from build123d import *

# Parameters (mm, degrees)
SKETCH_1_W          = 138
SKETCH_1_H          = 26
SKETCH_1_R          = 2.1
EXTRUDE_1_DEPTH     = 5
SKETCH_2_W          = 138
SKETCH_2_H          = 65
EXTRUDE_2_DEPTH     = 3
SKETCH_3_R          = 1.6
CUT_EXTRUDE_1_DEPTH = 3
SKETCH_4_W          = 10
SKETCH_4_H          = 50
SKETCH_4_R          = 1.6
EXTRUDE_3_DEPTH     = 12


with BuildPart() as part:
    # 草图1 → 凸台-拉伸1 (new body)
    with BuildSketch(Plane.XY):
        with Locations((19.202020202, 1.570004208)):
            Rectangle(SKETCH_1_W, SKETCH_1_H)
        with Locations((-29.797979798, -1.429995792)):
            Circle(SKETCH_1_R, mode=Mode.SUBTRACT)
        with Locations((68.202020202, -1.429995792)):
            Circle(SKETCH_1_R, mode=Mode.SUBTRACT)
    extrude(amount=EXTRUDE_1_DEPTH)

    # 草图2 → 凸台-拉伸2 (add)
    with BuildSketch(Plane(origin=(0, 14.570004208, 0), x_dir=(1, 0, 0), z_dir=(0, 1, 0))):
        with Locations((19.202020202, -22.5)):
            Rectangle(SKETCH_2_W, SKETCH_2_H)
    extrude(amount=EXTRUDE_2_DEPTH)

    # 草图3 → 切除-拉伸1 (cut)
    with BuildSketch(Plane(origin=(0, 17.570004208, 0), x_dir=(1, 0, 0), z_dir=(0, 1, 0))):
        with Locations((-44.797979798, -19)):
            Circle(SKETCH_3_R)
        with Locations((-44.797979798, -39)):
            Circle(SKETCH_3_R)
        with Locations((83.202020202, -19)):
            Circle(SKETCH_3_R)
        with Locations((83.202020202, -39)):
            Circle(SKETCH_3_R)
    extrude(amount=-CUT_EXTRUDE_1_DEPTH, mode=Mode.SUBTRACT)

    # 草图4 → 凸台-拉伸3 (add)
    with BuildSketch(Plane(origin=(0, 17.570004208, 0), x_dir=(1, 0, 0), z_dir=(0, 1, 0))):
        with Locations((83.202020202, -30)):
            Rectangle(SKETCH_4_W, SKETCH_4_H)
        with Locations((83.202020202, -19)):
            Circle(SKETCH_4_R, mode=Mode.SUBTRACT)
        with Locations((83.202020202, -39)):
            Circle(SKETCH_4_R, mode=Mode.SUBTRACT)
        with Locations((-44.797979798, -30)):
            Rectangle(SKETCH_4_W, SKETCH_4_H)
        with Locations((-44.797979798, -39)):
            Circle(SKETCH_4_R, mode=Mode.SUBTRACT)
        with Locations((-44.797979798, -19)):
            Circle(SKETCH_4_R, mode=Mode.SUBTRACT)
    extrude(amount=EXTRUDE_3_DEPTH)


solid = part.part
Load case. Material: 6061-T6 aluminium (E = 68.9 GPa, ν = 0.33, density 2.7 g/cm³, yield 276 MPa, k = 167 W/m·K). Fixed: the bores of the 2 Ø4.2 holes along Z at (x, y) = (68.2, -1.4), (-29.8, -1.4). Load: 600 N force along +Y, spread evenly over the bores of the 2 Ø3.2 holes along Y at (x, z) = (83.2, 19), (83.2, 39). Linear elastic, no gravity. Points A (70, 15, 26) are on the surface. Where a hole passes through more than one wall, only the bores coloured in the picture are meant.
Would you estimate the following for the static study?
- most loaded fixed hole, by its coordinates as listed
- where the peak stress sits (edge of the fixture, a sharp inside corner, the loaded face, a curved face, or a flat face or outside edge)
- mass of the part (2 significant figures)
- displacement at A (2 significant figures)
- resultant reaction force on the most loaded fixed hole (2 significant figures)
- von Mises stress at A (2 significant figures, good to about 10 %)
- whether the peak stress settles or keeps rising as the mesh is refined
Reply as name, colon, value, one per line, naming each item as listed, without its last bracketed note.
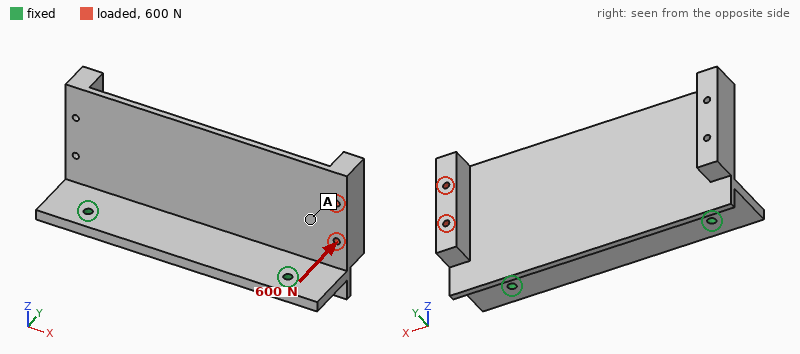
most loaded fixed hole, by its coordinates as listed: (68.2, -1.4)
where the peak stress sits: edge of the fixture
mass of the part: 150 g
displacement at A: 0.37 mm
resultant reaction force on the most loaded fixed hole: 690 N
von Mises stress at A: 18 MPa
whether the peak stress settles or keeps rising as the mesh is refined: keeps rising
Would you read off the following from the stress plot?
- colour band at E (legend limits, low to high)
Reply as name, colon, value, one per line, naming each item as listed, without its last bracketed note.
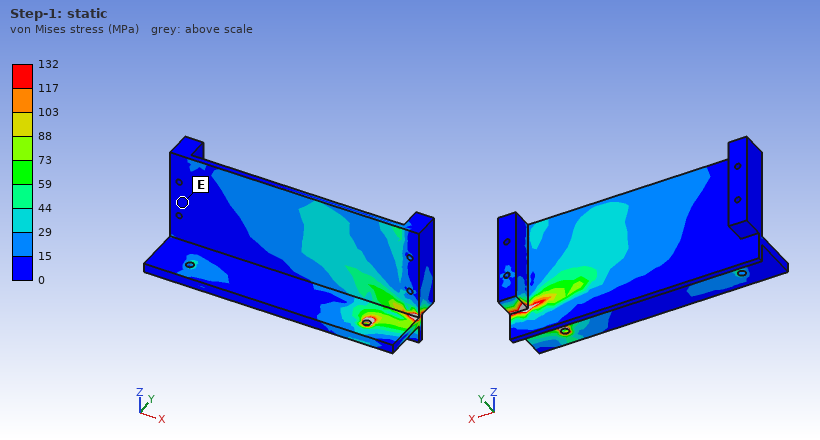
colour band at E: 0 to 15 MPa
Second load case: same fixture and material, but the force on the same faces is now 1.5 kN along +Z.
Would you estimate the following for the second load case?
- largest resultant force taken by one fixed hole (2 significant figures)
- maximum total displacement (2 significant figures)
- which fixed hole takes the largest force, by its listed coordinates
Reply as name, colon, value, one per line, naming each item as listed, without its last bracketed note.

largest resultant force taken by one fixed hole: 1.7 kN
maximum total displacement: 1.2 mm
which fixed hole takes the largest force, by its listed coordinates: (68.2, -1.4)
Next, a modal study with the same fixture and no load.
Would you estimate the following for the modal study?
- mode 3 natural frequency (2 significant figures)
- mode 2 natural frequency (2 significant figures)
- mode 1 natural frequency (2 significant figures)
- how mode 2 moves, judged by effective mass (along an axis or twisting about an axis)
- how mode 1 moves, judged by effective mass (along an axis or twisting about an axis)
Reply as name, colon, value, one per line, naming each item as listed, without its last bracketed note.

mode 3 natural frequency: 1800 Hz
mode 2 natural frequency: 870 Hz
mode 1 natural frequency: 700 Hz
how mode 2 moves, judged by effective mass: twisting about Z
how mode 1 moves, judged by effective mass: along Y
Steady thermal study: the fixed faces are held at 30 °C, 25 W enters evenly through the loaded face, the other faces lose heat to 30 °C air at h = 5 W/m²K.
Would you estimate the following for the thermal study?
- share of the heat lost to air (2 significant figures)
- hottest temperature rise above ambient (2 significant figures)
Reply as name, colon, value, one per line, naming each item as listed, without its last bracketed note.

share of the heat lost to air: 5.9 %
hottest temperature rise above ambient: 34 K
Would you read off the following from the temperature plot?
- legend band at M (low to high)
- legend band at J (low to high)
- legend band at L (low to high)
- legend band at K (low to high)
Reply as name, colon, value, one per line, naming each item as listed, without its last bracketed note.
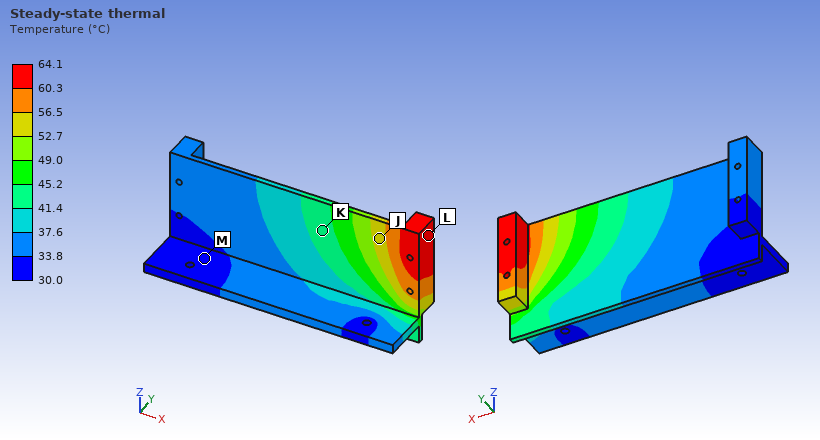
legend band at M: 30.0 to 33.8 °C
legend band at J: 52.7 to 56.5 °C
legend band at L: 60.3 to 64.1 °C
legend band at K: 41.4 to 45.2 °C
